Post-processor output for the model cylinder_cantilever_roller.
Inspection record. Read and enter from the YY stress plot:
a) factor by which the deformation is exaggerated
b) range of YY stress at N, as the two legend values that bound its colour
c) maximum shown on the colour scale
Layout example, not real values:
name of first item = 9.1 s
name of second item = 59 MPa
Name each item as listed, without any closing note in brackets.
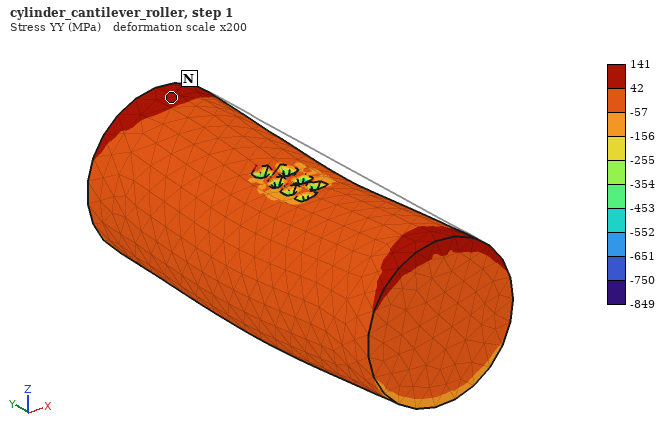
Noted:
factor by which the deformation is exaggerated = 200
range of YY stress at N, as the two legend values that bound its colour = 42 to 141 MPa
maximum shown on the colour scale = 141 MPa
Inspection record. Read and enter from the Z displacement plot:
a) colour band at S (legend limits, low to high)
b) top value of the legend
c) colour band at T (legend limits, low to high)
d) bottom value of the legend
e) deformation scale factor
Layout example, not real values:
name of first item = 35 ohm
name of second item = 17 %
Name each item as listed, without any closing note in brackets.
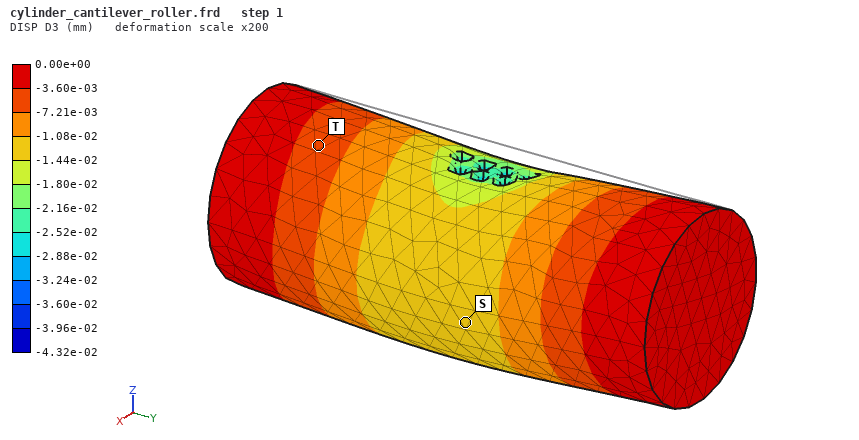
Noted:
colour band at S = -1.44e-02 to -1.08e-02 mm
top value of the legend = 0.00e+00 mm
colour band at T = -7.21e-03 to -3.60e-03 mm
bottom value of the legend = -4.32e-02 mm
deformation scale factor = 200
